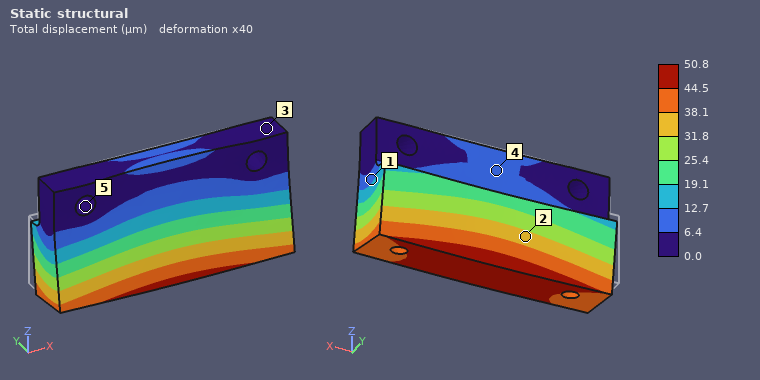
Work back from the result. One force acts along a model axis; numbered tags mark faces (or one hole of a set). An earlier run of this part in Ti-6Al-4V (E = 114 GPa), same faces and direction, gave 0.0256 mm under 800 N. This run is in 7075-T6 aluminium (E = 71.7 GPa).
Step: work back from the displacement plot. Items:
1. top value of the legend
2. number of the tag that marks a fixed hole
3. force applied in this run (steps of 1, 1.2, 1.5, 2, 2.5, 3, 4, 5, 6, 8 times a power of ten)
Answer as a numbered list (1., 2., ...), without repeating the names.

1. 50.8 µm
2. 5
3. 1 kN
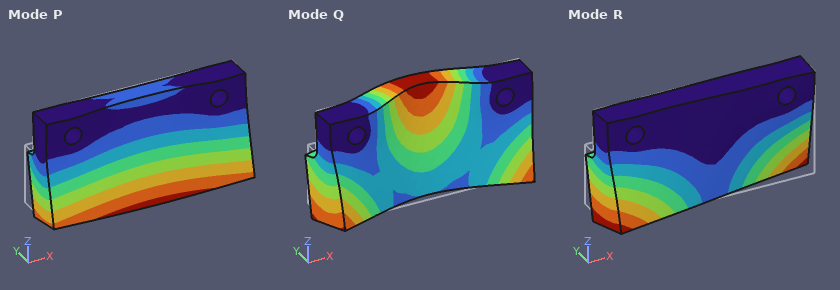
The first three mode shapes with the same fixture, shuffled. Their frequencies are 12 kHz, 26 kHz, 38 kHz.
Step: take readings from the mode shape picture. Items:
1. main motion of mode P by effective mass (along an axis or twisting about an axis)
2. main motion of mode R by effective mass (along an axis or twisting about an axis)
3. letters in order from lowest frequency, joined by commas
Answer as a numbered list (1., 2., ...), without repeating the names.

1. along Y
2. twisting about Z
3. P, R, Q
